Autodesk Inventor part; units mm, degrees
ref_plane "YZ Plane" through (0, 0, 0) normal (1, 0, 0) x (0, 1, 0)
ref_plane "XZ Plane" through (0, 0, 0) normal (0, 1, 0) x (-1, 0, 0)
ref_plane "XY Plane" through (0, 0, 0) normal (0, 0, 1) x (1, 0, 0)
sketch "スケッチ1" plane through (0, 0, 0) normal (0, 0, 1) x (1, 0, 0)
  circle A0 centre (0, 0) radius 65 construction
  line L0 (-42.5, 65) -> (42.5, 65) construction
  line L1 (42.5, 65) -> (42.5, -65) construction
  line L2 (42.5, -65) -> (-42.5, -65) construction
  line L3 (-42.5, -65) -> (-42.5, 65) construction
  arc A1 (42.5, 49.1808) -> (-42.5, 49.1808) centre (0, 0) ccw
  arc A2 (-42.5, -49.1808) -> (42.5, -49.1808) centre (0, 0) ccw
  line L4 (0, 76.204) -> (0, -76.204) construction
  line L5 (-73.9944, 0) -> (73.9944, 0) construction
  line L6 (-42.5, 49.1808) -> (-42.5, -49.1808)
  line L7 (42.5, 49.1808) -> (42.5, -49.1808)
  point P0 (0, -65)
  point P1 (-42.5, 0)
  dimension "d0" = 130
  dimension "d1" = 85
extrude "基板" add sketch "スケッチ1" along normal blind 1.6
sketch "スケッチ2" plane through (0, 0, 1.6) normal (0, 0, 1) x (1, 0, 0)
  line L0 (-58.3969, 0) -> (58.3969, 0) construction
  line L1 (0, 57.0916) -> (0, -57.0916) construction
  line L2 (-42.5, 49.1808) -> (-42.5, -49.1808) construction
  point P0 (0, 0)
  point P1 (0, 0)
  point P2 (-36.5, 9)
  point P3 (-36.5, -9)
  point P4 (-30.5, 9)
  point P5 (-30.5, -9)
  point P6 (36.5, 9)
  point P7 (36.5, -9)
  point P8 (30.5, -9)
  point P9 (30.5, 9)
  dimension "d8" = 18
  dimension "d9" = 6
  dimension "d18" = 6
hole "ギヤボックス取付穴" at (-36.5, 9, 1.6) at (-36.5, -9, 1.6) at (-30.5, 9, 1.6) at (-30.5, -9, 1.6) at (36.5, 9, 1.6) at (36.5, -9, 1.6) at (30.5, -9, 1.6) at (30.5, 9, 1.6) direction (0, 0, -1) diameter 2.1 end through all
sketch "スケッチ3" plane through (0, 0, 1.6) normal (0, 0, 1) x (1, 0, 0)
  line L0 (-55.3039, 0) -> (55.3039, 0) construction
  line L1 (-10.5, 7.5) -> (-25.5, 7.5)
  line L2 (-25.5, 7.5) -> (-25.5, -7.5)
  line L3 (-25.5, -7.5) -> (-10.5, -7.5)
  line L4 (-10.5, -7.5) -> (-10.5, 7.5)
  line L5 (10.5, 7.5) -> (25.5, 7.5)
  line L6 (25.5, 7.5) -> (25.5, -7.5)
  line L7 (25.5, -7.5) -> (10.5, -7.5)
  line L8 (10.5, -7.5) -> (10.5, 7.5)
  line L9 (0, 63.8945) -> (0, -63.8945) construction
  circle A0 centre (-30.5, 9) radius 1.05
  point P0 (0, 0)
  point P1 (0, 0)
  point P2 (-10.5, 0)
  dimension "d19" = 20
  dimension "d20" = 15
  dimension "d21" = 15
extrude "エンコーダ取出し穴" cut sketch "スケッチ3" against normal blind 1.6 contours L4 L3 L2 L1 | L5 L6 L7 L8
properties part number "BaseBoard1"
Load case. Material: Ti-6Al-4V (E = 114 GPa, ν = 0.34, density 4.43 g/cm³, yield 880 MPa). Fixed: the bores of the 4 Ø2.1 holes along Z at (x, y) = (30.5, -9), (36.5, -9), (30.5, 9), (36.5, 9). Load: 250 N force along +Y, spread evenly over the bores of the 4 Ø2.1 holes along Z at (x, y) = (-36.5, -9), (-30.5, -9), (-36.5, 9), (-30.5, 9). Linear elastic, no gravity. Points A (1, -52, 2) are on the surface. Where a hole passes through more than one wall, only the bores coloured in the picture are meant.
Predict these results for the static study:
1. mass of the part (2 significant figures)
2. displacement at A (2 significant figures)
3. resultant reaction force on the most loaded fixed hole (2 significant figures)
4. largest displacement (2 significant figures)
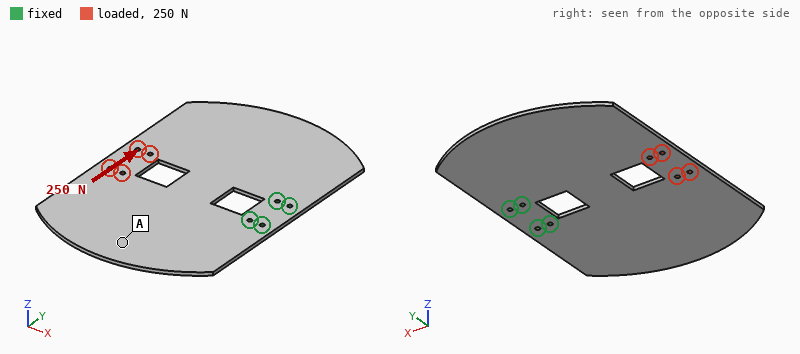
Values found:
69 g
42 µm
560 N
65 µm
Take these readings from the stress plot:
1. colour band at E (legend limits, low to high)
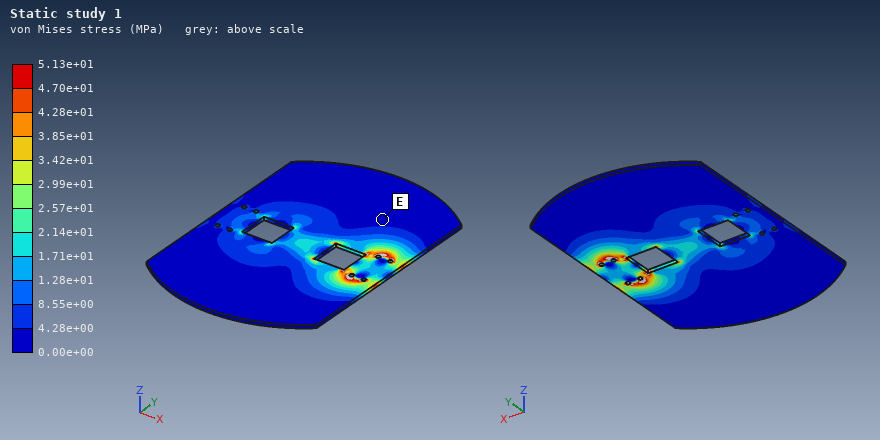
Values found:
0.00e+00 to 4.28e+00 MPa
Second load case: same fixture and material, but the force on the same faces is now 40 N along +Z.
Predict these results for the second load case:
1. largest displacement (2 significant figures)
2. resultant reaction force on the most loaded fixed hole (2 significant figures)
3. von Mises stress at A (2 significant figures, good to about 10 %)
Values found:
1.8 mm
130 N
22 MPa
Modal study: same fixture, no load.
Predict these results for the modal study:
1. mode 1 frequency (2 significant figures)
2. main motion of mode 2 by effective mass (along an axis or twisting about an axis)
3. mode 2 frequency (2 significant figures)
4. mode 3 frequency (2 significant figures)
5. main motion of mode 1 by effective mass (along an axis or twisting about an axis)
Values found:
170 Hz
twisting about X
230 Hz
470 Hz
along Z
